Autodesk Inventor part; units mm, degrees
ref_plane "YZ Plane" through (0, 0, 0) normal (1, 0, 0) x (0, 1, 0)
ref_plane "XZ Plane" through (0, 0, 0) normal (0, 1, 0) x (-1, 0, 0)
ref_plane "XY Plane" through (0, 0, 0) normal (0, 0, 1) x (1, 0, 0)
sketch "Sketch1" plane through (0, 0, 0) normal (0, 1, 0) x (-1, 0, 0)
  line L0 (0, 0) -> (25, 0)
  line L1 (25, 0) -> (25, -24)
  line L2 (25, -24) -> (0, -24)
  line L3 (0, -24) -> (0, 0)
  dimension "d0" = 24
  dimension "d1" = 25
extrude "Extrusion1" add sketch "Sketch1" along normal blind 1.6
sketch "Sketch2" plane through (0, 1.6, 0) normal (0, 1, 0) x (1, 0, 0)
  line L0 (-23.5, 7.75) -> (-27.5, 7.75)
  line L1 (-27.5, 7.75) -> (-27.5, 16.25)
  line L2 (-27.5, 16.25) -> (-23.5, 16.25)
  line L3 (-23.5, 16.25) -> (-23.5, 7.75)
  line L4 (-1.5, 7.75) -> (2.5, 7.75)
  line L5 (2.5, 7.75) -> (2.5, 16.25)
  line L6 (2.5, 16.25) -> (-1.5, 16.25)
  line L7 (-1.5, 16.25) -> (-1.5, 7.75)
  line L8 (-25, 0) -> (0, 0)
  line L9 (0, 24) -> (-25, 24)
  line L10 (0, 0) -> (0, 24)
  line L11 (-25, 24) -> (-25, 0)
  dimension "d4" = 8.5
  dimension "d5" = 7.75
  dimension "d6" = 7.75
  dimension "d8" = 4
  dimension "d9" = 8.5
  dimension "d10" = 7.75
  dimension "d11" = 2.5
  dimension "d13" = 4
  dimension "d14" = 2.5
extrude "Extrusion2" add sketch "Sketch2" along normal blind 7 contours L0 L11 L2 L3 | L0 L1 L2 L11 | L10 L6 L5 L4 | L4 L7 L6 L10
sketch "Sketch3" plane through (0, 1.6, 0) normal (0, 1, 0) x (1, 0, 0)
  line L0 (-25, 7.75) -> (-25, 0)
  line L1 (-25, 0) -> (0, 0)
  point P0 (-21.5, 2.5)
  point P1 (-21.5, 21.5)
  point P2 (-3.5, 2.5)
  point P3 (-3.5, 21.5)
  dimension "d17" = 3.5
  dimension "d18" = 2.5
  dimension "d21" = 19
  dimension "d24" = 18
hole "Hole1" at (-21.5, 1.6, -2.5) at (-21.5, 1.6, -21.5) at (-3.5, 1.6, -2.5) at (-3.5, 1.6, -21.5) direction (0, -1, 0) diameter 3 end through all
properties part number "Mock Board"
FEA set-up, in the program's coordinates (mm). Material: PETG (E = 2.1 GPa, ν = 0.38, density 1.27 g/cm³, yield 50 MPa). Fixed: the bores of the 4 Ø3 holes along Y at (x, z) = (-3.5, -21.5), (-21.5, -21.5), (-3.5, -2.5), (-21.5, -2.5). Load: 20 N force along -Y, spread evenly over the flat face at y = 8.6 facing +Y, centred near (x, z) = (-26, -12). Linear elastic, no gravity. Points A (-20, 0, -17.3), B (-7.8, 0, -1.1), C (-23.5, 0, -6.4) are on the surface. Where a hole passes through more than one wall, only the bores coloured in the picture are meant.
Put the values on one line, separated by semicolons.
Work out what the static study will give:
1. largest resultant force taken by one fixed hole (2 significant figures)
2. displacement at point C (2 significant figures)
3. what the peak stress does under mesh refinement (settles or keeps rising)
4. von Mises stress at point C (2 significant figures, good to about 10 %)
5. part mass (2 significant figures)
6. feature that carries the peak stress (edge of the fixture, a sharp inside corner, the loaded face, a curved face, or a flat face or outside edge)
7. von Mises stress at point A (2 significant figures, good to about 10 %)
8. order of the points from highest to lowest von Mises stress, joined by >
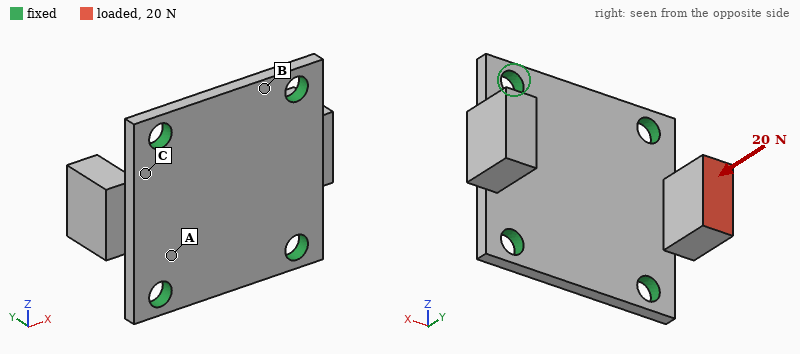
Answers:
12 N; 0.047 mm; keeps rising; 9.4 MPa; 1.8 g; edge of the fixture; 5.0 MPa; C > A > B
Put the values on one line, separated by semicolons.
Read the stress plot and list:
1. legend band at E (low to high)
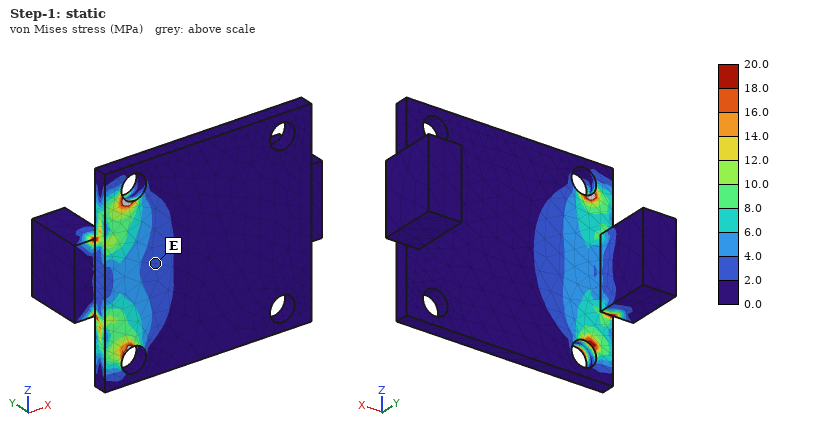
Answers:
2.0 to 4.0 MPa
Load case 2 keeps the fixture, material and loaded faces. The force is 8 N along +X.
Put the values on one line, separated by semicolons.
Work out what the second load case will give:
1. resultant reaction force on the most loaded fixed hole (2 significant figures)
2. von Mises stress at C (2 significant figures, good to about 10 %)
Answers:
2.6 N; 8.0 MPa
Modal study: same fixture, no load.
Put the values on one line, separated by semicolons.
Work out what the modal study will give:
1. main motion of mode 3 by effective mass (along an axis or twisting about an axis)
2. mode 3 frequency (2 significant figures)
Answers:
along Y; 4900 Hz
